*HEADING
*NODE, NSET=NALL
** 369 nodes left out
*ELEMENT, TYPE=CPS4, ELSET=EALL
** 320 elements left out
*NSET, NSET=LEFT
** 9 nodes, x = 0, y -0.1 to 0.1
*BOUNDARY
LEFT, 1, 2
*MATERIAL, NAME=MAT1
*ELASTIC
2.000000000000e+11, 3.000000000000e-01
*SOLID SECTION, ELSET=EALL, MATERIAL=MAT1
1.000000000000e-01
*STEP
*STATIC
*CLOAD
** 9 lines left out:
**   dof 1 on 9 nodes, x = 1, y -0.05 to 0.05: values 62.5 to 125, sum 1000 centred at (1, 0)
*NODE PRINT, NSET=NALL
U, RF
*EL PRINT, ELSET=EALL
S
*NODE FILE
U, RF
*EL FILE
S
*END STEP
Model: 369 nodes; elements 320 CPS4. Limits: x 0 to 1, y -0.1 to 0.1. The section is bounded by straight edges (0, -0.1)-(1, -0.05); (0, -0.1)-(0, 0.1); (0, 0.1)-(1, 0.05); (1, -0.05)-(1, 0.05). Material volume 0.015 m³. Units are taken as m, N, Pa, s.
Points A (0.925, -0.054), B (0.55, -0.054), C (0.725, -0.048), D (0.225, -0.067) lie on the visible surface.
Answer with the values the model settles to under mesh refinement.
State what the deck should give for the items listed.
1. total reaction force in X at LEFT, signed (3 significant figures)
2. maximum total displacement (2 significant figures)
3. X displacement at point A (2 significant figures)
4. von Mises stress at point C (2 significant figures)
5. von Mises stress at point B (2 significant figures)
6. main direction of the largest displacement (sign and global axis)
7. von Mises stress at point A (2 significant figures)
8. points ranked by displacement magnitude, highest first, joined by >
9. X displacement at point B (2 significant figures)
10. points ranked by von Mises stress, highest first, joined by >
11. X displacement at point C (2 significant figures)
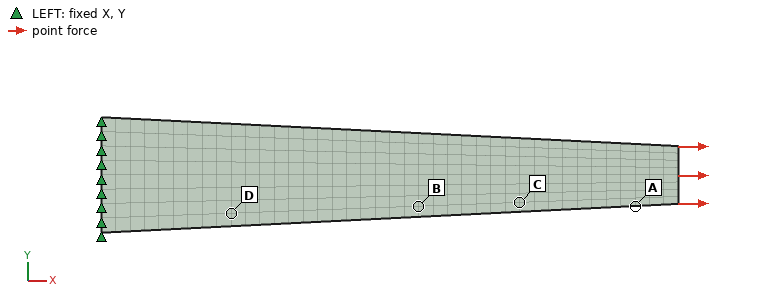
-1000 N
3.5e-07 m
3.1e-07 m
78000 Pa
69000 Pa
+X
93000 Pa
A > C > B > D
1.6e-07 m
A > C > B > D
2.2e-07 m
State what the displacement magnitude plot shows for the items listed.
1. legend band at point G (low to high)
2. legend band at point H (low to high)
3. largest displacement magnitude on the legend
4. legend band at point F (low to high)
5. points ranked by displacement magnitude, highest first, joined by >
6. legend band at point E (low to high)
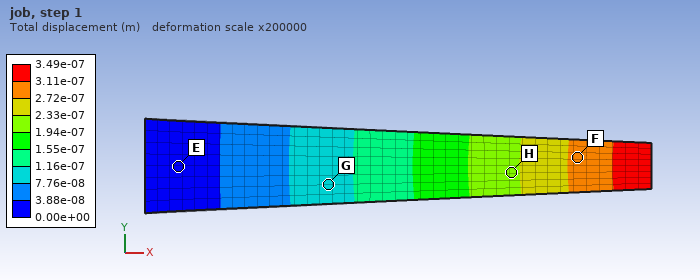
7.76e-08 to 1.16e-07 m
1.94e-07 to 2.33e-07 m
3.49e-07 m
2.72e-07 to 3.11e-07 m
F > H > G > E
0.00e+00 to 3.88e-08 m
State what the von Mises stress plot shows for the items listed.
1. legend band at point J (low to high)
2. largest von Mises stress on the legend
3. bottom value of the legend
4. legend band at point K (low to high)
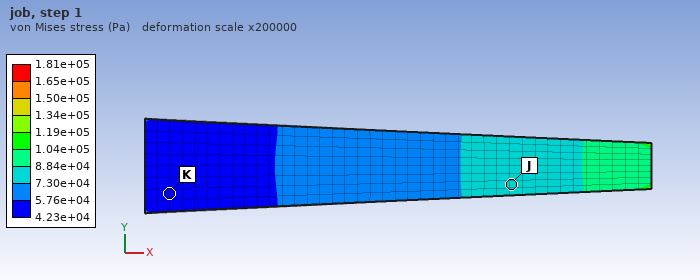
7.30e+04 to 8.84e+04 Pa
1.81e+05 Pa
4.23e+04 Pa
4.23e+04 to 5.76e+04 Pa
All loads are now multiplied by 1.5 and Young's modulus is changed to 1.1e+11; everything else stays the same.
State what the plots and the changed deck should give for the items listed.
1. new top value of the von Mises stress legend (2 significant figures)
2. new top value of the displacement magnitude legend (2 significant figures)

2.7e+05 Pa
9.5e-07 m
